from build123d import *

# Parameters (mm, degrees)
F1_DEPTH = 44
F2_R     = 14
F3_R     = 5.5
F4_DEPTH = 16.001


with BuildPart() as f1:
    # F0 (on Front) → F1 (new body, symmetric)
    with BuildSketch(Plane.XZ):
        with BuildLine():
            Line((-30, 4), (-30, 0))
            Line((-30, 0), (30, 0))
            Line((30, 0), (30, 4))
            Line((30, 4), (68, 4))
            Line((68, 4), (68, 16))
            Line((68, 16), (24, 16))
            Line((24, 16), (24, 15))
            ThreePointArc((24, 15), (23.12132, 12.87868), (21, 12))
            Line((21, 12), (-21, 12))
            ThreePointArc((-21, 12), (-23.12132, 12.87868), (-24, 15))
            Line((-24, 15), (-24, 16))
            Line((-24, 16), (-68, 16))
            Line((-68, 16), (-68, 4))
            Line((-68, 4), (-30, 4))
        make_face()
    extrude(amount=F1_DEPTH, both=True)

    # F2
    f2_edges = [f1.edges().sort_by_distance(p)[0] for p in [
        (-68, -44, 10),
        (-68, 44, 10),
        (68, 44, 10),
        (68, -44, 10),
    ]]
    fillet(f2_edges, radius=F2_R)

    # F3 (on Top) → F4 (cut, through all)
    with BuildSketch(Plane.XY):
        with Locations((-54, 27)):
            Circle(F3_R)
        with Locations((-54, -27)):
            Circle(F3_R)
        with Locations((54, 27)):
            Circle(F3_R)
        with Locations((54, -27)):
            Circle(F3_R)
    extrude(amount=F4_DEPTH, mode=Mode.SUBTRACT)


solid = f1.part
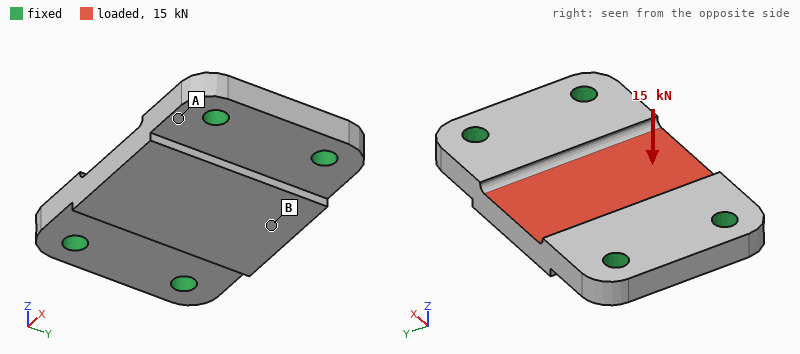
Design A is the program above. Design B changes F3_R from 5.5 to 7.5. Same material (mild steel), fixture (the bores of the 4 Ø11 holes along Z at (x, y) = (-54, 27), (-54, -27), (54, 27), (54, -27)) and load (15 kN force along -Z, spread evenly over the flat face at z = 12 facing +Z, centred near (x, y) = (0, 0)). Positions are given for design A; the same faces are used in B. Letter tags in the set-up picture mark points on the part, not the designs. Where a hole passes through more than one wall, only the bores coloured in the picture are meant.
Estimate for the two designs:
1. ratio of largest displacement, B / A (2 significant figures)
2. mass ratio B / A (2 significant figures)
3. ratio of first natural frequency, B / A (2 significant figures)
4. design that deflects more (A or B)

0.85
0.97
1.1
A
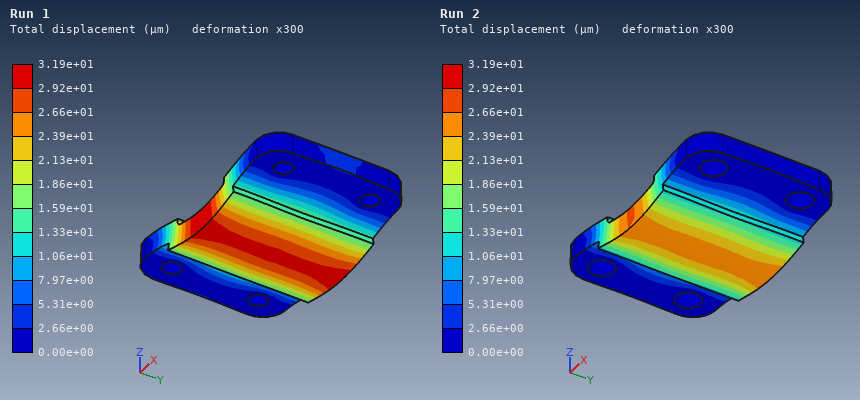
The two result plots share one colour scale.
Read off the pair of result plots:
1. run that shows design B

Run 2
